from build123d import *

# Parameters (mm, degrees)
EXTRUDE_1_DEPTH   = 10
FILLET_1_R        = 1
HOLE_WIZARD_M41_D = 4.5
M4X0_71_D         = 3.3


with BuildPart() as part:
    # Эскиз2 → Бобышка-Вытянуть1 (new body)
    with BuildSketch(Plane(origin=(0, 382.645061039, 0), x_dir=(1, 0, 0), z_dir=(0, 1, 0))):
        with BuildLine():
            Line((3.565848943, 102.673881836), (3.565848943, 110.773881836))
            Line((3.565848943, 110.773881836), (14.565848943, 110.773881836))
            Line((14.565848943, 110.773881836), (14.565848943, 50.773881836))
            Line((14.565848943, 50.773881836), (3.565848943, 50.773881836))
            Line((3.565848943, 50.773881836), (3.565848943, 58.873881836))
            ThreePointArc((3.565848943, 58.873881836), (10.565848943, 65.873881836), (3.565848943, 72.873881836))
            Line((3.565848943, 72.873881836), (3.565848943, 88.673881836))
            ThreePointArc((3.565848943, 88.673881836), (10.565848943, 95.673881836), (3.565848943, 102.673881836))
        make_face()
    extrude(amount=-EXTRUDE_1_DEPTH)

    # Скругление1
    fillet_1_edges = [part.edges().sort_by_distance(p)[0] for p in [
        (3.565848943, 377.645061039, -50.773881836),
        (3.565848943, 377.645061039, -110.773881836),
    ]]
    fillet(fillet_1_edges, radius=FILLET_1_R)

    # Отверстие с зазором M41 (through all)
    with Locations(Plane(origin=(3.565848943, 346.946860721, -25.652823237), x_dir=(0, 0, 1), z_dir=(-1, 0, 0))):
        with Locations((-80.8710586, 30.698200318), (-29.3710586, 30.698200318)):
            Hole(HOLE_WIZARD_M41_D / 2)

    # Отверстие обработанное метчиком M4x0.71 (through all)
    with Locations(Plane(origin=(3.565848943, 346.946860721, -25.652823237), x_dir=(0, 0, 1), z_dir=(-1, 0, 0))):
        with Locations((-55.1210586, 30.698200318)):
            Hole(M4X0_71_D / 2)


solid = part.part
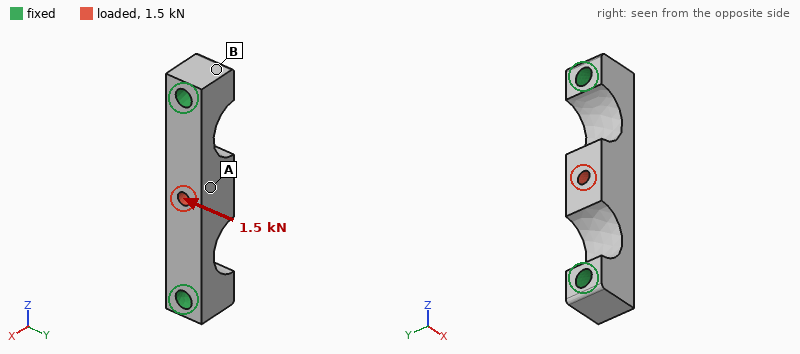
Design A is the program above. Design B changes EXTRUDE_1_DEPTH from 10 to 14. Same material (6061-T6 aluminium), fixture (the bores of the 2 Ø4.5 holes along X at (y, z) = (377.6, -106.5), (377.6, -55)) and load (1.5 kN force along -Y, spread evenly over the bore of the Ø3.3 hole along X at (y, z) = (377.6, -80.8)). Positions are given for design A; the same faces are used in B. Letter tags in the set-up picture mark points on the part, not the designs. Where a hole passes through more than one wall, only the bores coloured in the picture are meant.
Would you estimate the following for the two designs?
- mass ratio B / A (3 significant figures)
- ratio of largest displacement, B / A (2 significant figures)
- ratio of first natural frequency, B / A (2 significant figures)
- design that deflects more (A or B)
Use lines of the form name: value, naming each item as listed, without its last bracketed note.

mass ratio B / A: 1.44
ratio of largest displacement, B / A: 0.58
ratio of first natural frequency, B / A: 1.0
design that deflects more: A
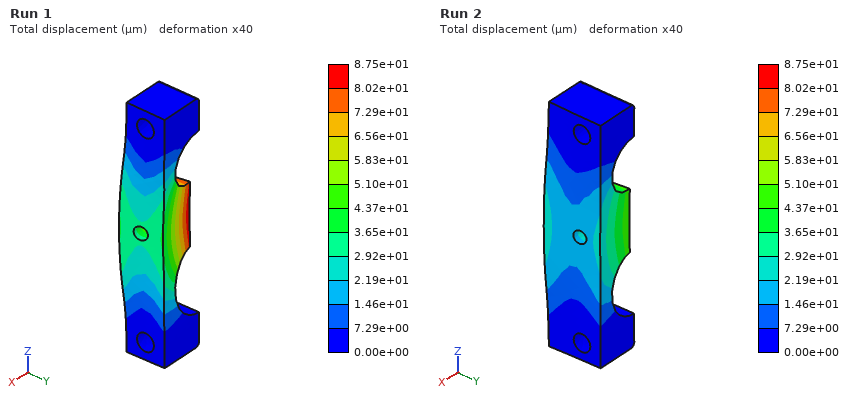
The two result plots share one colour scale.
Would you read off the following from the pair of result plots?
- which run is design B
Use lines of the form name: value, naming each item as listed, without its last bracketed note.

which run is design B: Run 2
